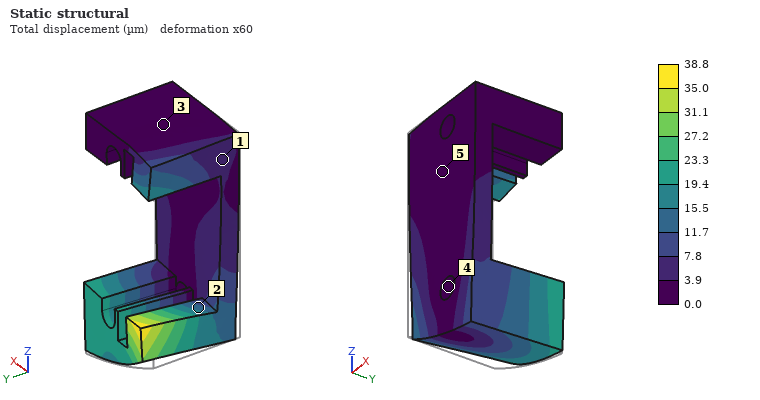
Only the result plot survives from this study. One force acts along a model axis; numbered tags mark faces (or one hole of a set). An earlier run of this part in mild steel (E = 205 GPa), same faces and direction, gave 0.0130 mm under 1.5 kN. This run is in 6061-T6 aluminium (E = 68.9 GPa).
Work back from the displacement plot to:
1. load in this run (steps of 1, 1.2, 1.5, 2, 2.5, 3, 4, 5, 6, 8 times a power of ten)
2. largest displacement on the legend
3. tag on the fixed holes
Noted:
1.5 kN
38.8 µm
4
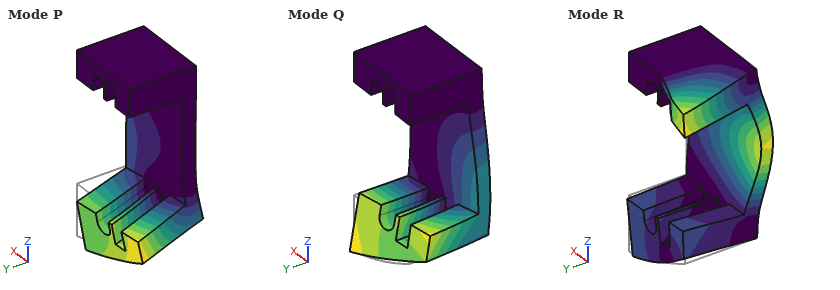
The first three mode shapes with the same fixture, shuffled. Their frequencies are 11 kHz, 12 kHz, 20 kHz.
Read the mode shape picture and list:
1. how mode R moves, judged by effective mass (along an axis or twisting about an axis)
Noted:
along Y
